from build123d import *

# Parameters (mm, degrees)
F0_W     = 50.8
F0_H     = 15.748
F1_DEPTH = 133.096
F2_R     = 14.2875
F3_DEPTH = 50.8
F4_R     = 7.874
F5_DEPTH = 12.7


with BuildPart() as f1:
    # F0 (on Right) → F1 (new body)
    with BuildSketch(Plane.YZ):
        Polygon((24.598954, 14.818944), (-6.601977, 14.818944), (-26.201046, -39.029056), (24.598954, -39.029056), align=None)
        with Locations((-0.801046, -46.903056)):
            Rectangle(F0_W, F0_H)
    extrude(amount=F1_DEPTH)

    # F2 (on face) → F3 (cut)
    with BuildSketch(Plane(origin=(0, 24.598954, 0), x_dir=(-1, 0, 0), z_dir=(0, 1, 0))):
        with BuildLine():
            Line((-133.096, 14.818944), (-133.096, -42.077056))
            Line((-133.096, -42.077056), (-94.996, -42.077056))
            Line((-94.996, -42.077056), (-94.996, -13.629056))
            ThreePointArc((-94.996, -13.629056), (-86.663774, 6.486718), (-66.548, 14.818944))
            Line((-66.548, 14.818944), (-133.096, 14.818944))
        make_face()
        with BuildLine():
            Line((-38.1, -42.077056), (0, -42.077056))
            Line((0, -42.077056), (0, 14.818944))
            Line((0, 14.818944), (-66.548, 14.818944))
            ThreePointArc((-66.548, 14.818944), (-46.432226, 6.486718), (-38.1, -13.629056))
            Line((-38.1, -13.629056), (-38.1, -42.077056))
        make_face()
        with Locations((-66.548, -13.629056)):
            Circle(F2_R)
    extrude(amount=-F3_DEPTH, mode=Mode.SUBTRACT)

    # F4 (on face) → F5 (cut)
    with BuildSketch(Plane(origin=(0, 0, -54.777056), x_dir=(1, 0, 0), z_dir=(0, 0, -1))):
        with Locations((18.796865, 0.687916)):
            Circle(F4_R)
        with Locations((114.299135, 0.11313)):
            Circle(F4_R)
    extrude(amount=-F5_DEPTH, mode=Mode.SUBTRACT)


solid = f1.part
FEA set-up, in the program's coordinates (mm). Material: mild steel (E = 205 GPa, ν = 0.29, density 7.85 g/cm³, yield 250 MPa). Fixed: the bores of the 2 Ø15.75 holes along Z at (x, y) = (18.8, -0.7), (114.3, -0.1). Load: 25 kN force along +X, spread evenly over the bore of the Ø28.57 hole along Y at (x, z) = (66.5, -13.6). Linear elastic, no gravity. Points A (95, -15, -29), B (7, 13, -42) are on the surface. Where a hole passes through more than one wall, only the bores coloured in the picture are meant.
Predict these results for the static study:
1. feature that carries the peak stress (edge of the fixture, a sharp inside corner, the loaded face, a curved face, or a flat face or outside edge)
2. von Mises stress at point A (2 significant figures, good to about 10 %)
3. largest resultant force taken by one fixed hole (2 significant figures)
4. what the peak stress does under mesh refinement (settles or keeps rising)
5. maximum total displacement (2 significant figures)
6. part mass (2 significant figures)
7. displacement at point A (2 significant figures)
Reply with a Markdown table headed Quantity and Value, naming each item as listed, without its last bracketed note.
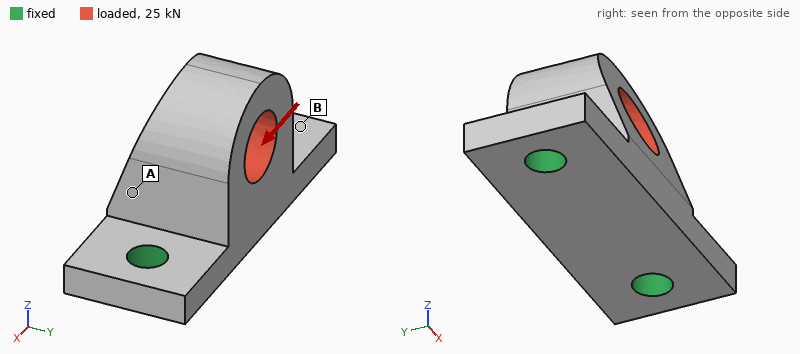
| Quantity | Value |
|---|---|
| feature that carries the peak stress | edge of the fixture |
| von Mises stress at point A | 36 MPa |
| largest resultant force taken by one fixed hole | 17 kN |
| what the peak stress does under mesh refinement | keeps rising |
| maximum total displacement | 38 µm |
| part mass | 1.4 kg |
| displacement at point A | 16 µm |
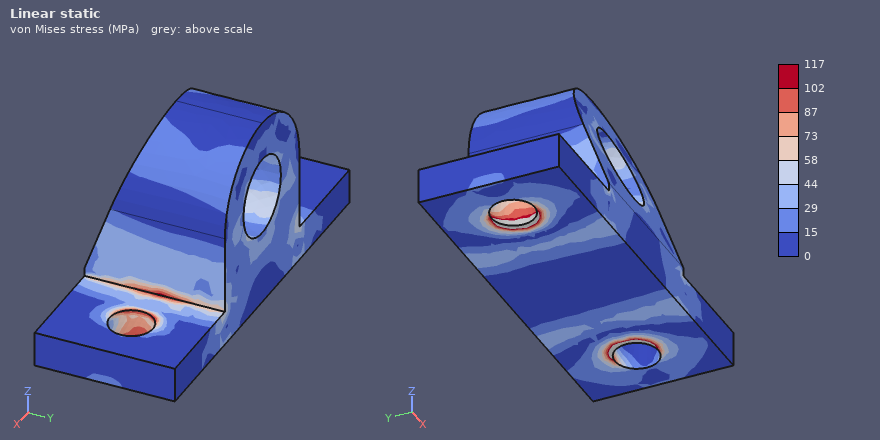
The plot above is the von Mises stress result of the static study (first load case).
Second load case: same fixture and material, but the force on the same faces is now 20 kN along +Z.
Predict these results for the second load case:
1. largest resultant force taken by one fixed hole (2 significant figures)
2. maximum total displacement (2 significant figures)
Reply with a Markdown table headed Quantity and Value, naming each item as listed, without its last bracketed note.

| Quantity | Value |
|---|---|
| largest resultant force taken by one fixed hole | 11 kN |
| maximum total displacement | 26 µm |
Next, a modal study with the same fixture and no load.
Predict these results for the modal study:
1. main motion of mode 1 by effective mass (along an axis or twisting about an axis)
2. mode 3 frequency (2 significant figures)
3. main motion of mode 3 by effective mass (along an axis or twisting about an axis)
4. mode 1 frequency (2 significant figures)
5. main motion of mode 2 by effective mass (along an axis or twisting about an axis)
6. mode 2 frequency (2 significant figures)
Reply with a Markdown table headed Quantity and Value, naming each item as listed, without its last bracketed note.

| Quantity | Value |
|---|---|
| main motion of mode 1 by effective mass | along Y |
| mode 3 frequency | 6200 Hz |
| main motion of mode 3 by effective mass | along Z |
| mode 1 frequency | 2700 Hz |
| main motion of mode 2 by effective mass | along X |
| mode 2 frequency | 5800 Hz |
